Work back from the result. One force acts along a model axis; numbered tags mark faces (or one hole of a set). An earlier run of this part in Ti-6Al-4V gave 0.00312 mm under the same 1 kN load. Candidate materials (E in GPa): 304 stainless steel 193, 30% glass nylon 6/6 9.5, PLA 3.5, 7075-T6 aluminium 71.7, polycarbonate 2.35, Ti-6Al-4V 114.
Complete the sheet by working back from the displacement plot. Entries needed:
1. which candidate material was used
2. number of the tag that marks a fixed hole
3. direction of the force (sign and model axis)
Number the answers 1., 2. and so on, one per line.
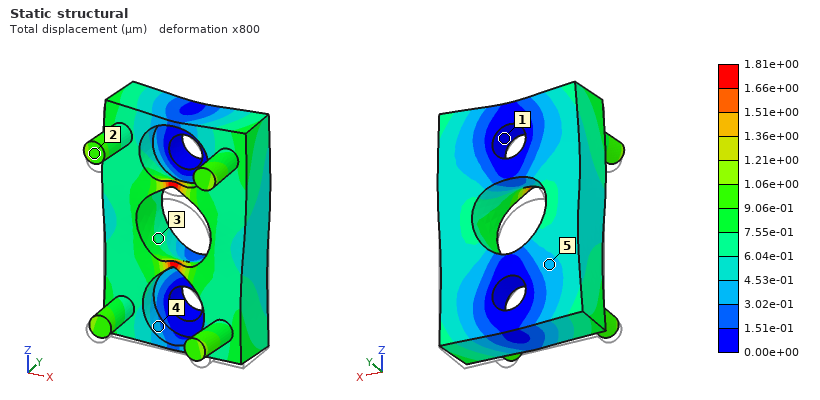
1. 304 stainless steel
2. 1
3. +Z
